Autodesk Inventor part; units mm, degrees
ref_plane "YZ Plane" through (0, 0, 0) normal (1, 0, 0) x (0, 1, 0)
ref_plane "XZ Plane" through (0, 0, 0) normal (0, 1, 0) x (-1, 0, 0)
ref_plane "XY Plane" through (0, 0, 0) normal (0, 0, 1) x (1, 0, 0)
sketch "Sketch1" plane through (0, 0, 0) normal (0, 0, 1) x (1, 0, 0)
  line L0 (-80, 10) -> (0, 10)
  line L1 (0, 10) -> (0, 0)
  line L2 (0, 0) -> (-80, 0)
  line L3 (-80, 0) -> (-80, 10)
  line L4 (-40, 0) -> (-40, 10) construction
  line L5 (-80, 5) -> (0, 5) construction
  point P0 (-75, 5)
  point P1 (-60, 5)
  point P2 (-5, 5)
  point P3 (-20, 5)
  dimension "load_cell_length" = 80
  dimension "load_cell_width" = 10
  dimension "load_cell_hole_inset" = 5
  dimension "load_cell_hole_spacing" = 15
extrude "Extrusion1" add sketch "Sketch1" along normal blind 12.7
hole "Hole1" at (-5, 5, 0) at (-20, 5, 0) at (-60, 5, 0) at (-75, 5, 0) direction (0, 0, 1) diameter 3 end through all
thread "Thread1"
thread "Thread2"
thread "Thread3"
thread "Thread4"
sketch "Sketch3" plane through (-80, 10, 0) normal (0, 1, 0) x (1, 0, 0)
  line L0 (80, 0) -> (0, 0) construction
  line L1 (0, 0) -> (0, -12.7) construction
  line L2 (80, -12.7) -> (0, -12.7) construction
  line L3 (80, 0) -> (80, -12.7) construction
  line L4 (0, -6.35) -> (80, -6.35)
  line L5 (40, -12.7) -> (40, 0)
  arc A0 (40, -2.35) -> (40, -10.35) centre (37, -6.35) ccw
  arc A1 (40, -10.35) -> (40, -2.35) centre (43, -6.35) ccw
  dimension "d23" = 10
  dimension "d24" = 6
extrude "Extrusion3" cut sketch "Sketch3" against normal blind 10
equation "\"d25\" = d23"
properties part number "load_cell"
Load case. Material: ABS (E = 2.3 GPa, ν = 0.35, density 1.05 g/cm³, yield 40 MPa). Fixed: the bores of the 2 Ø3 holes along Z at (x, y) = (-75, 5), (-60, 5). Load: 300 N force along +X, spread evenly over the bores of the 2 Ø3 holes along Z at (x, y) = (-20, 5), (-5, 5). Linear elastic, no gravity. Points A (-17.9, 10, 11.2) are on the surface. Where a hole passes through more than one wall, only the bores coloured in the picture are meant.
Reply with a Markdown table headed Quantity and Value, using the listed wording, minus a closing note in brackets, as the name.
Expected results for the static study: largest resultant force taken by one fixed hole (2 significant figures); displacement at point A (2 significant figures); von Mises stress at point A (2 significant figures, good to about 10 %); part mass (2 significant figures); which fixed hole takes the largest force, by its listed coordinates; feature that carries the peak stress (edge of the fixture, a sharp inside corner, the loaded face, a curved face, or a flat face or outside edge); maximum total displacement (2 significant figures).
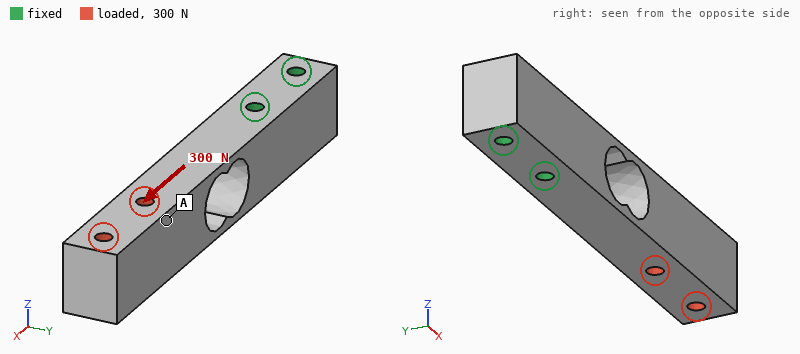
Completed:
| Quantity | Value |
|---|---|
| largest resultant force taken by one fixed hole | 270 N |
| displacement at point A | 0.11 mm |
| von Mises stress at point A | 2.1 MPa |
| part mass | 8.9 g |
| which fixed hole takes the largest force, by its listed coordinates | (-60, 5) |
| feature that carries the peak stress | a curved face |
| maximum total displacement | 0.12 mm |
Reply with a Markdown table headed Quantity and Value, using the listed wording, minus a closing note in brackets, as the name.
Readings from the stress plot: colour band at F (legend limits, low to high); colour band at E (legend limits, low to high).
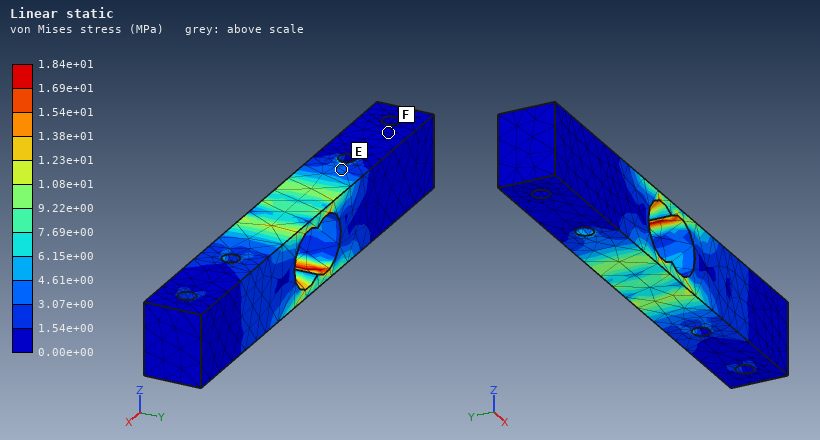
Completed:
| Quantity | Value |
|---|---|
| colour band at F | 0.00e+00 to 1.54e+00 MPa |
| colour band at E | 3.07e+00 to 4.61e+00 MPa |
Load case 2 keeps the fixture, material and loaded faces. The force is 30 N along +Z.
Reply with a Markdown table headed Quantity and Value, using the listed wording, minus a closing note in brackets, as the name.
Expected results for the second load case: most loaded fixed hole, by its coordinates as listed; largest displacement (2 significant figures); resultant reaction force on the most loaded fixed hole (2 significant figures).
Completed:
| Quantity | Value |
|---|---|
| most loaded fixed hole, by its coordinates as listed | (-60, 5) |
| largest displacement | 0.87 mm |
| resultant reaction force on the most loaded fixed hole | 42 N |
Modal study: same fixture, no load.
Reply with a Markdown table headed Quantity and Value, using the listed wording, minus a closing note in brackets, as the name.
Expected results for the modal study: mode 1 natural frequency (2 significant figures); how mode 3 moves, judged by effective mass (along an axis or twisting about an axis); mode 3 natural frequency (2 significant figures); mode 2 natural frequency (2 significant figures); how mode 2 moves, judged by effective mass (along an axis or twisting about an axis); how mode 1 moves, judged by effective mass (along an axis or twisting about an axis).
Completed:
| Quantity | Value |
|---|---|
| mode 1 natural frequency | 440 Hz |
| how mode 3 moves, judged by effective mass | twisting about X |
| mode 3 natural frequency | 2100 Hz |
| mode 2 natural frequency | 520 Hz |
| how mode 2 moves, judged by effective mass | along Z |
| how mode 1 moves, judged by effective mass | along Y |
